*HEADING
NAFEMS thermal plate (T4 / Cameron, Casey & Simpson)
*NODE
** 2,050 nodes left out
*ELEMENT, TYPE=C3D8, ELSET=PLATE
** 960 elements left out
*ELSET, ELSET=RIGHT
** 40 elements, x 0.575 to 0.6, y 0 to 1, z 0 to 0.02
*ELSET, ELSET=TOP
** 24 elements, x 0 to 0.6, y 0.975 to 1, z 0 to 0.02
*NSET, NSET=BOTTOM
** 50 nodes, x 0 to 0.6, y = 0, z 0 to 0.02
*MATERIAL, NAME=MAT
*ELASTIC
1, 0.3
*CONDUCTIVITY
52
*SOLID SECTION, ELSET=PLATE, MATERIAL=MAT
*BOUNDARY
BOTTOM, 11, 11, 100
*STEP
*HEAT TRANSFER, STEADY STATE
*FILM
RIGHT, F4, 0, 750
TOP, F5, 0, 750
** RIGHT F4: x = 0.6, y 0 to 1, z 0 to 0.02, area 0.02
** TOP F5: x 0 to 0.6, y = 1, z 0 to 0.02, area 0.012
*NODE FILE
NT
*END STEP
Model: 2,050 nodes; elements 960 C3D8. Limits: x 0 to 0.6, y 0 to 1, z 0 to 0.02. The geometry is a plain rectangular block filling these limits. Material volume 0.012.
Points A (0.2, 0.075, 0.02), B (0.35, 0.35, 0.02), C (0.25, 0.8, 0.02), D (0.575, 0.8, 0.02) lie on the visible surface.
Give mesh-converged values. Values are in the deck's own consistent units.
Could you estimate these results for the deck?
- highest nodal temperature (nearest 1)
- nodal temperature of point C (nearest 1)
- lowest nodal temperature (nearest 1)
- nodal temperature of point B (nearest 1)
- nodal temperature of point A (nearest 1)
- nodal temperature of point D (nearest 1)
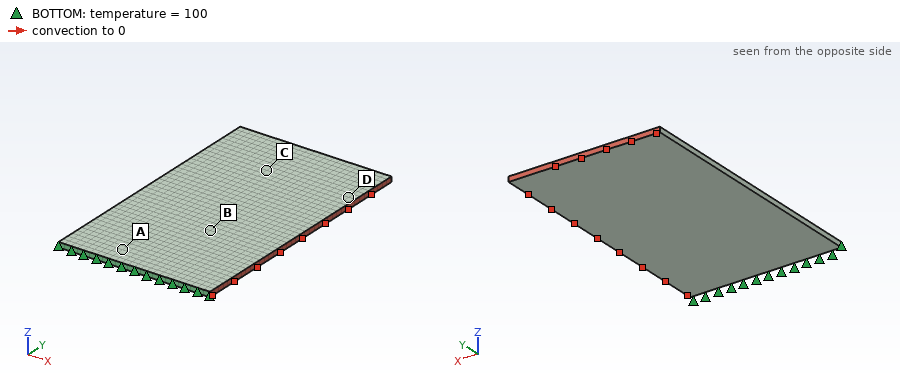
100
12
1
39
87
3
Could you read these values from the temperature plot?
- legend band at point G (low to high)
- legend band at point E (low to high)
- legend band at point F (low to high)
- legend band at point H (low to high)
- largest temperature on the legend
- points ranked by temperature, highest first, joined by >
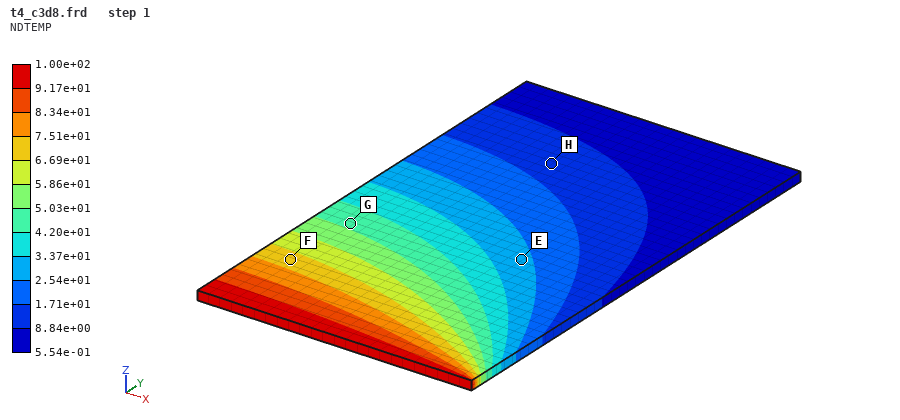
4.20e+01 to 5.03e+01
2.54e+01 to 3.37e+01
6.69e+01 to 7.51e+01
8.84e+00 to 1.71e+01
1.00e+02
F > G > E > H
